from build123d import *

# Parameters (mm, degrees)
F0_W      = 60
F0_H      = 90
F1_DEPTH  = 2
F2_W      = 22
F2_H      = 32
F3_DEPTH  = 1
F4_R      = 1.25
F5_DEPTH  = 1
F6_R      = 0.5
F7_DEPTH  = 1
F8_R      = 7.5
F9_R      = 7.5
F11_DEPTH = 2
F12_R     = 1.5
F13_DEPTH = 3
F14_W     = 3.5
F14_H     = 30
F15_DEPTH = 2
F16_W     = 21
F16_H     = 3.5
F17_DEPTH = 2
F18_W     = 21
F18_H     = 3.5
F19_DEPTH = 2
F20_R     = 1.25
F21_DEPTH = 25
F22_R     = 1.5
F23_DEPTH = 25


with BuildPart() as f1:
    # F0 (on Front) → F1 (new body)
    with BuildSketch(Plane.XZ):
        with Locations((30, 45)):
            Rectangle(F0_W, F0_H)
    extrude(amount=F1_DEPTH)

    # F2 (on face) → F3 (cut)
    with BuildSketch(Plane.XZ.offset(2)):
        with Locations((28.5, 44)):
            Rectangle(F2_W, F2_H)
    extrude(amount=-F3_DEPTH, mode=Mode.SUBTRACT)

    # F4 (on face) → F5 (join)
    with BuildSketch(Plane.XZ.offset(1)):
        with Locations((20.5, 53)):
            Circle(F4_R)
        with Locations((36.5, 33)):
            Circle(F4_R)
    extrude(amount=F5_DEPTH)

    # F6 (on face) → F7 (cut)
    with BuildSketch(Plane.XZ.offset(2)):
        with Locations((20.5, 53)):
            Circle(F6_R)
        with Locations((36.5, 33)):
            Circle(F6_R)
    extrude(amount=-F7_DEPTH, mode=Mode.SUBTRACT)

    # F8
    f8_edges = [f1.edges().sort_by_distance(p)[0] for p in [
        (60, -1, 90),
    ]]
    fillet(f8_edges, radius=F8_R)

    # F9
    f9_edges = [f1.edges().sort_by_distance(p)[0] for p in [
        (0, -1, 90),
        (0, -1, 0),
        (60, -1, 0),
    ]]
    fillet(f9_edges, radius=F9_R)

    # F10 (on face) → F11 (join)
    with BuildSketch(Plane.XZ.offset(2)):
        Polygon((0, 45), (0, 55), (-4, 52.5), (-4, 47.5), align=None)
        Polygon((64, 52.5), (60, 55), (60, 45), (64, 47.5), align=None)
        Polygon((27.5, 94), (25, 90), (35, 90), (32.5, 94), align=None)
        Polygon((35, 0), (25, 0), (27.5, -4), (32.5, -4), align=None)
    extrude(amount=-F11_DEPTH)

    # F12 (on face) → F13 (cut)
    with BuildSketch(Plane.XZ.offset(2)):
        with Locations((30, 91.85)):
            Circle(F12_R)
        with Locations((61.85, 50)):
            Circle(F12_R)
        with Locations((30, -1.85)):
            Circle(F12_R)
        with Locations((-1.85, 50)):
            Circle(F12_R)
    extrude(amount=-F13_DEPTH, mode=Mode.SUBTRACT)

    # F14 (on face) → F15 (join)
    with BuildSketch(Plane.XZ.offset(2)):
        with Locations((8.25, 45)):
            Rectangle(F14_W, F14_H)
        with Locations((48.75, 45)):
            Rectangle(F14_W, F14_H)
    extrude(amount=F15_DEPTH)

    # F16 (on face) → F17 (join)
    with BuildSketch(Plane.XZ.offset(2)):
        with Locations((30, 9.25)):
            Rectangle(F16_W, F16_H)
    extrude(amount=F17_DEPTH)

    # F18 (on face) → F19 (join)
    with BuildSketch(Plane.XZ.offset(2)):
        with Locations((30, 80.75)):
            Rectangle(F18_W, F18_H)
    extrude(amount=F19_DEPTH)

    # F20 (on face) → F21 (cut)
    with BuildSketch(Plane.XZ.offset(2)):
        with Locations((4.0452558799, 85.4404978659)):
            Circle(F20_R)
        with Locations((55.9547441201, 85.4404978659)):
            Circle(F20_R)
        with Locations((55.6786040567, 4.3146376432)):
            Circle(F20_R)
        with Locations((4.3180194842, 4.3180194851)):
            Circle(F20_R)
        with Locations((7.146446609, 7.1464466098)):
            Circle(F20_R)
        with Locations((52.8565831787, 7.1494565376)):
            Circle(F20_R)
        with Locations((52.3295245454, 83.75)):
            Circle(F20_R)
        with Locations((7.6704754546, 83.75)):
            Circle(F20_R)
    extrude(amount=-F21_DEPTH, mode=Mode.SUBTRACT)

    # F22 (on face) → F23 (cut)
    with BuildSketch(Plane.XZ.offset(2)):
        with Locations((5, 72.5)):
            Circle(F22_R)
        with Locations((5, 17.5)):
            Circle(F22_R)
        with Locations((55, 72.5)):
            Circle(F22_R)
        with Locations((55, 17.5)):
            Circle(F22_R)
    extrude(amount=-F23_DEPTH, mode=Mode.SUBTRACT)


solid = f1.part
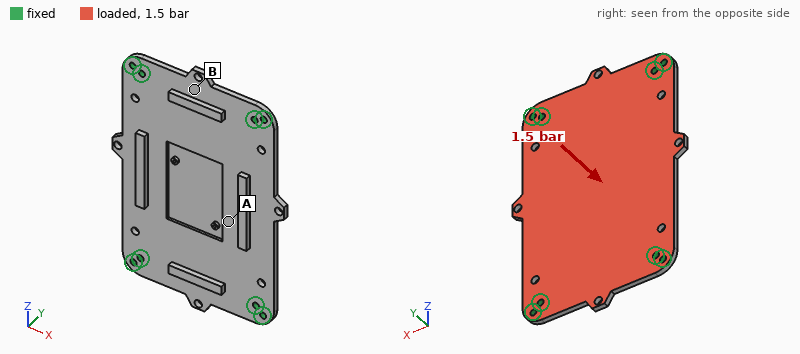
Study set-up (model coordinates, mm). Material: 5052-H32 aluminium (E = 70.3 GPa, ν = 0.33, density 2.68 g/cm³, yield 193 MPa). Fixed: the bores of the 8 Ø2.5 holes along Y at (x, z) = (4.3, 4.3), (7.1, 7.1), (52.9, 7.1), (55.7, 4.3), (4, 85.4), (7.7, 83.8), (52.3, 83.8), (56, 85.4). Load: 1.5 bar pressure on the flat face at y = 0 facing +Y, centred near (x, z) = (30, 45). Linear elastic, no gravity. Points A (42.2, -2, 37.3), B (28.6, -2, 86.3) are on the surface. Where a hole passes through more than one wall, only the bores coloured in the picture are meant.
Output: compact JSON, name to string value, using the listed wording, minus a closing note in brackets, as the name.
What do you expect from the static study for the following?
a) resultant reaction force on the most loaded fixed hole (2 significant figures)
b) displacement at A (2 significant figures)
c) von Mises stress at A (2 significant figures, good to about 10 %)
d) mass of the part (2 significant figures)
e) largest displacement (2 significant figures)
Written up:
{"resultant reaction force on the most loaded fixed hole": "330 N", "displacement at A": "0.30 mm", "von Mises stress at A": "35 MPa", "mass of the part": "29 g", "largest displacement": "0.37 mm"}
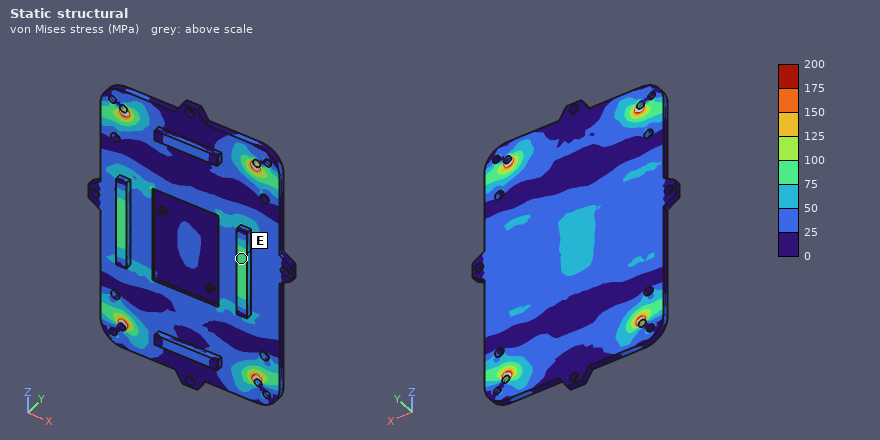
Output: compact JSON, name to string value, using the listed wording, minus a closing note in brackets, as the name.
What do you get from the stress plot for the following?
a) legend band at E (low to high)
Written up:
{"legend band at E": "75 to 100 MPa"}
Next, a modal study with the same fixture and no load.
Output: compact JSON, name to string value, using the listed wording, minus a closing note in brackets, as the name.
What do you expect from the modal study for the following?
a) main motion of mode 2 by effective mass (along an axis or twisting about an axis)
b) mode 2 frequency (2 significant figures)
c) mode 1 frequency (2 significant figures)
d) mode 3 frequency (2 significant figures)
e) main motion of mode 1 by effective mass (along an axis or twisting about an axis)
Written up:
{"main motion of mode 2 by effective mass": "twisting about Z", "mode 2 frequency": "2400 Hz", "mode 1 frequency": "1800 Hz", "mode 3 frequency": "3700 Hz", "main motion of mode 1 by effective mass": "along Y"}
